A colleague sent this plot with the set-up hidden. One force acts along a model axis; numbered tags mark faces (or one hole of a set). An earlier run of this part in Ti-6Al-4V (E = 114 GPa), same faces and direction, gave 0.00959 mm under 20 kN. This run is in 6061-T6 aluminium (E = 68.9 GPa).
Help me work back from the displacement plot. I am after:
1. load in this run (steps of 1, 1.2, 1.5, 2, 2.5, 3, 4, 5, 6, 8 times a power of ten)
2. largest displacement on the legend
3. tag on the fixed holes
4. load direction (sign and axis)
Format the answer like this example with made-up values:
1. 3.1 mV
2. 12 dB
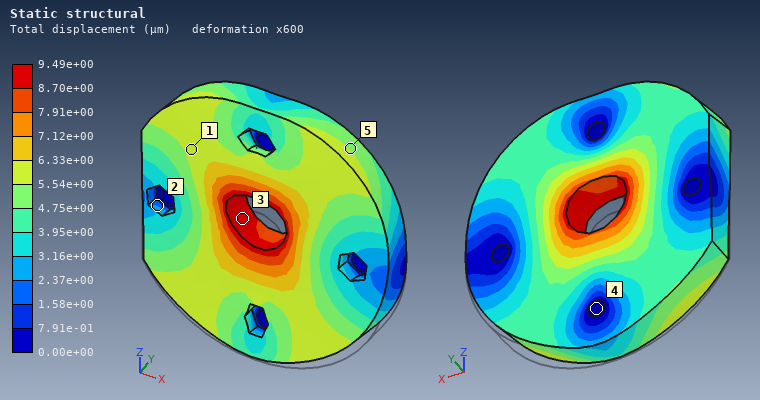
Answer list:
1. 12 kN
2. 9.49e+00 µm
3. 4
4. +Z
